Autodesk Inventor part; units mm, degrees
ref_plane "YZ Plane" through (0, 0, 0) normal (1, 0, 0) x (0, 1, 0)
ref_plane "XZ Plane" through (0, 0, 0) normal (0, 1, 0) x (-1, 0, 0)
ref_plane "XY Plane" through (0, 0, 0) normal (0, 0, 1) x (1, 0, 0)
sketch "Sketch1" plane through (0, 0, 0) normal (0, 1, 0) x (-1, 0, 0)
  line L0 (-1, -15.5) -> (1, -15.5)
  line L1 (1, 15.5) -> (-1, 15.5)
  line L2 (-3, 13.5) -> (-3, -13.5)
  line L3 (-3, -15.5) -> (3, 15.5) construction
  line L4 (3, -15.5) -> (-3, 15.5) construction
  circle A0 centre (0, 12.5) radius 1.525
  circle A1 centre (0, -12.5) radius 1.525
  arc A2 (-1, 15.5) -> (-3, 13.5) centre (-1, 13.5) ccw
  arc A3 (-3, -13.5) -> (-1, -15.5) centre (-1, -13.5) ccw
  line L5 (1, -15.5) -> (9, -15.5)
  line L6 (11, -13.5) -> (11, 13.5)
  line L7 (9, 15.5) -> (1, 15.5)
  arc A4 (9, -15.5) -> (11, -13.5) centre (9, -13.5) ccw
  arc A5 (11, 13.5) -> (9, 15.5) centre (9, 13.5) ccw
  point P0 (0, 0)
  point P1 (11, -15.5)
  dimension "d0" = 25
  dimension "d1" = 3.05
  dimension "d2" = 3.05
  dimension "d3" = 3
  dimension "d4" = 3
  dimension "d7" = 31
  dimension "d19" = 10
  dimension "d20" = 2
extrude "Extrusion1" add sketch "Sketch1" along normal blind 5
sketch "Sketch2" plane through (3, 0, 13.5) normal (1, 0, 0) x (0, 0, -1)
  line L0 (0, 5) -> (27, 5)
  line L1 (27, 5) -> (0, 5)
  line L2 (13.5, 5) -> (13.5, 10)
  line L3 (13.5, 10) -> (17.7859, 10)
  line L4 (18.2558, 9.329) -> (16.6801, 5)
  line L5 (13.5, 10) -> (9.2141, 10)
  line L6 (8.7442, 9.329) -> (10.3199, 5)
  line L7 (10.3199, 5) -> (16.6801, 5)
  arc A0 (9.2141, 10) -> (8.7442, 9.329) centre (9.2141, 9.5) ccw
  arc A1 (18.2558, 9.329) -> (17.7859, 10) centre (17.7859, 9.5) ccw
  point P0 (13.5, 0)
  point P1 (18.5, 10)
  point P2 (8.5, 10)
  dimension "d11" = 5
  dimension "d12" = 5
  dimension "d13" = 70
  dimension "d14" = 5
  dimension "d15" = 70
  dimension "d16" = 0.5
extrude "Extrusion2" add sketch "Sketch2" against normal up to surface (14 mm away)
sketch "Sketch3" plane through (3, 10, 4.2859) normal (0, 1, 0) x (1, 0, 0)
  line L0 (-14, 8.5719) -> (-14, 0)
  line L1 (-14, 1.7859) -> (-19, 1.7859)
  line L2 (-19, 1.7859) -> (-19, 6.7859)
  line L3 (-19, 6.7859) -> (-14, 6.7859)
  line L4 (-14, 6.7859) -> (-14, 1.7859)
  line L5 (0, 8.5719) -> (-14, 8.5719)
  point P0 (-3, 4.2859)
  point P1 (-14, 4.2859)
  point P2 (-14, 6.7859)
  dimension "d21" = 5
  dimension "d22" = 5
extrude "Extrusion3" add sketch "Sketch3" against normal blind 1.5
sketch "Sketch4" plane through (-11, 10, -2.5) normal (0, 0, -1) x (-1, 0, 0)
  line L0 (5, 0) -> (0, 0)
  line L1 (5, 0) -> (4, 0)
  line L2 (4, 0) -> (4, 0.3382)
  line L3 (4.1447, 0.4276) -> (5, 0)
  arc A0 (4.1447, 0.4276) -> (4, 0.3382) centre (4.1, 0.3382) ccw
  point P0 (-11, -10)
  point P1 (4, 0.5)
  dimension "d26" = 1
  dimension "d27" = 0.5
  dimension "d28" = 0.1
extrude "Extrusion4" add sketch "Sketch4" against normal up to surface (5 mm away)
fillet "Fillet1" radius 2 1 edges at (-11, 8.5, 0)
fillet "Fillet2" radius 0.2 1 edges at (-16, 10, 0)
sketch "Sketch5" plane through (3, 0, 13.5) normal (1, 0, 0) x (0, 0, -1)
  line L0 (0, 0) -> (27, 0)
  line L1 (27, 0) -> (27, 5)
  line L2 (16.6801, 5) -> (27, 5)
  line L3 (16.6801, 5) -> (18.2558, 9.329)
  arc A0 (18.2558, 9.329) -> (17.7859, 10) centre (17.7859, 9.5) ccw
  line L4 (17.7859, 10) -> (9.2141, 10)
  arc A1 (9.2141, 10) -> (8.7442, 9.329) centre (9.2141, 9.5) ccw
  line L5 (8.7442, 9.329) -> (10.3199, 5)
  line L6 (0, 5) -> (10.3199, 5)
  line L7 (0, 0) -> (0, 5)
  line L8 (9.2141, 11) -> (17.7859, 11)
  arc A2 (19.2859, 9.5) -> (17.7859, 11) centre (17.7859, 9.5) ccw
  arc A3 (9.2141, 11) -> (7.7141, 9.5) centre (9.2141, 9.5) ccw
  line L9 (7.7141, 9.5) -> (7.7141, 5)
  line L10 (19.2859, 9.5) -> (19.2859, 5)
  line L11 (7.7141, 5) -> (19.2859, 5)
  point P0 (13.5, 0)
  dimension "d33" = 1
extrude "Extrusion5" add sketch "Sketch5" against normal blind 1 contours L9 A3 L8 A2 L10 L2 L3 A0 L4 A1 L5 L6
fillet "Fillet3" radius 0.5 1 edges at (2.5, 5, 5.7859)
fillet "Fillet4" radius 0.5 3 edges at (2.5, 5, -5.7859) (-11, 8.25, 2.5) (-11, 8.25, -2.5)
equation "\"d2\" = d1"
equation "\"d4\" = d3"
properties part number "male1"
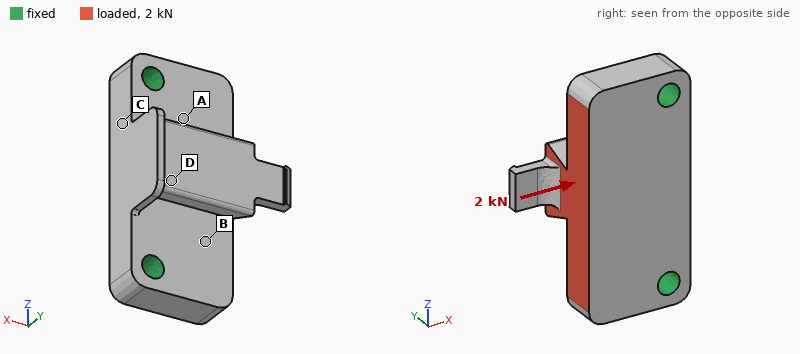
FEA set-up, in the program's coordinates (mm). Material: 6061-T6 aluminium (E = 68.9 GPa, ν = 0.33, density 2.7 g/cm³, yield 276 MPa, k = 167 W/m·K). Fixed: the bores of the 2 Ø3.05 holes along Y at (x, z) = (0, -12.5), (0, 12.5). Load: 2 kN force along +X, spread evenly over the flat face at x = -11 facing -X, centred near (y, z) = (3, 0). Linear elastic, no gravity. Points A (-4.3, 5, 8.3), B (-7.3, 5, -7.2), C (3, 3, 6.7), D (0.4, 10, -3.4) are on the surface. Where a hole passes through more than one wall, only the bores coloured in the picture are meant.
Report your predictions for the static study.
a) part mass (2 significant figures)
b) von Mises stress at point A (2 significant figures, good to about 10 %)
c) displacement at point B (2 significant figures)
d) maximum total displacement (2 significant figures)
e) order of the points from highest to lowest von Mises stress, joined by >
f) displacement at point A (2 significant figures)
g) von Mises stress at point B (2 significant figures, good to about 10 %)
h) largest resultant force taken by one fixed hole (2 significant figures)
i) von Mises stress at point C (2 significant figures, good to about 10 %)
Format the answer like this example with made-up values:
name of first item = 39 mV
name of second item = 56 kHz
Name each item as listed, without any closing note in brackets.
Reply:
part mass = 7.3 g
von Mises stress at point A = 35 MPa
displacement at point B = 6.2 µm
maximum total displacement = 14 µm
order of the points from highest to lowest von Mises stress, joined by > = A > B > C > D
displacement at point A = 4.4 µm
von Mises stress at point B = 24 MPa
largest resultant force taken by one fixed hole = 1.1 kN
von Mises stress at point C = 16 MPa
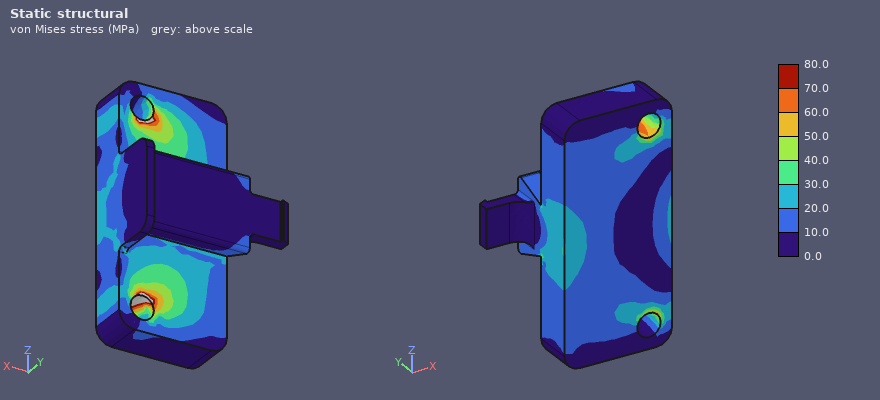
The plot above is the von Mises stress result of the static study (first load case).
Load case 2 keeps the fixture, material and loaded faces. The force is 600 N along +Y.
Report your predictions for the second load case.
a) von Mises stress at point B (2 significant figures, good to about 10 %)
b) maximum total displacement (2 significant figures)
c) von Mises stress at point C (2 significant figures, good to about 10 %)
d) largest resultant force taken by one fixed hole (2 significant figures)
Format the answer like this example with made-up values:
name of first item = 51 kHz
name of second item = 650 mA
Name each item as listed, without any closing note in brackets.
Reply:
von Mises stress at point B = 21 MPa
maximum total displacement = 41 µm
von Mises stress at point C = 30 MPa
largest resultant force taken by one fixed hole = 300 N
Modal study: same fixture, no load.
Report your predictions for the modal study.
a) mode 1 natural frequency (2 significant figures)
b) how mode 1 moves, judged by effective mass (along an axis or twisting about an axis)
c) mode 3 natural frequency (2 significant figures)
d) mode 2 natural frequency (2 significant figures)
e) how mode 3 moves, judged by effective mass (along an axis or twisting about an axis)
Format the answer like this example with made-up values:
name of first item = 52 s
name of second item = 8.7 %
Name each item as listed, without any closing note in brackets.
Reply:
mode 1 natural frequency = 15 kHz
how mode 1 moves, judged by effective mass = along Y
mode 3 natural frequency = 34 kHz
mode 2 natural frequency = 28 kHz
how mode 3 moves, judged by effective mass = along Z
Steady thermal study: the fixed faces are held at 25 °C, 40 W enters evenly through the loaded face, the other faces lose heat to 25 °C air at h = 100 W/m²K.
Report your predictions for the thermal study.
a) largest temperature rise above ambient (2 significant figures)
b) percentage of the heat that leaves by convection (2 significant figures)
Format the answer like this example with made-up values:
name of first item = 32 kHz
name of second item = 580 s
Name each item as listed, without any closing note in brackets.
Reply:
largest temperature rise above ambient = 23 K
percentage of the heat that leaves by convection = 4.4 %
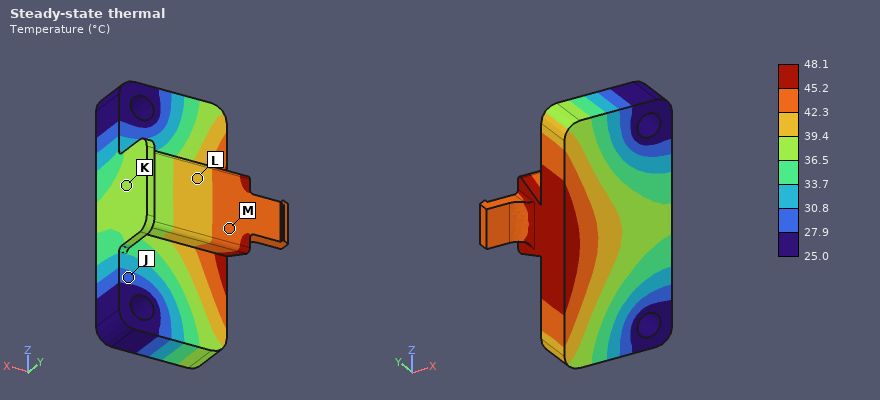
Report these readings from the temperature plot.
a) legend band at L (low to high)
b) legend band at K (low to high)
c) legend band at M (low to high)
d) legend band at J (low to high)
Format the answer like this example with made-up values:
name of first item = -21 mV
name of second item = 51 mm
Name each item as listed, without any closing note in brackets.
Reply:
legend band at L = 39.4 to 42.3 °C
legend band at K = 36.5 to 39.4 °C
legend band at M = 42.3 to 45.2 °C
legend band at J = 27.9 to 30.8 °C
